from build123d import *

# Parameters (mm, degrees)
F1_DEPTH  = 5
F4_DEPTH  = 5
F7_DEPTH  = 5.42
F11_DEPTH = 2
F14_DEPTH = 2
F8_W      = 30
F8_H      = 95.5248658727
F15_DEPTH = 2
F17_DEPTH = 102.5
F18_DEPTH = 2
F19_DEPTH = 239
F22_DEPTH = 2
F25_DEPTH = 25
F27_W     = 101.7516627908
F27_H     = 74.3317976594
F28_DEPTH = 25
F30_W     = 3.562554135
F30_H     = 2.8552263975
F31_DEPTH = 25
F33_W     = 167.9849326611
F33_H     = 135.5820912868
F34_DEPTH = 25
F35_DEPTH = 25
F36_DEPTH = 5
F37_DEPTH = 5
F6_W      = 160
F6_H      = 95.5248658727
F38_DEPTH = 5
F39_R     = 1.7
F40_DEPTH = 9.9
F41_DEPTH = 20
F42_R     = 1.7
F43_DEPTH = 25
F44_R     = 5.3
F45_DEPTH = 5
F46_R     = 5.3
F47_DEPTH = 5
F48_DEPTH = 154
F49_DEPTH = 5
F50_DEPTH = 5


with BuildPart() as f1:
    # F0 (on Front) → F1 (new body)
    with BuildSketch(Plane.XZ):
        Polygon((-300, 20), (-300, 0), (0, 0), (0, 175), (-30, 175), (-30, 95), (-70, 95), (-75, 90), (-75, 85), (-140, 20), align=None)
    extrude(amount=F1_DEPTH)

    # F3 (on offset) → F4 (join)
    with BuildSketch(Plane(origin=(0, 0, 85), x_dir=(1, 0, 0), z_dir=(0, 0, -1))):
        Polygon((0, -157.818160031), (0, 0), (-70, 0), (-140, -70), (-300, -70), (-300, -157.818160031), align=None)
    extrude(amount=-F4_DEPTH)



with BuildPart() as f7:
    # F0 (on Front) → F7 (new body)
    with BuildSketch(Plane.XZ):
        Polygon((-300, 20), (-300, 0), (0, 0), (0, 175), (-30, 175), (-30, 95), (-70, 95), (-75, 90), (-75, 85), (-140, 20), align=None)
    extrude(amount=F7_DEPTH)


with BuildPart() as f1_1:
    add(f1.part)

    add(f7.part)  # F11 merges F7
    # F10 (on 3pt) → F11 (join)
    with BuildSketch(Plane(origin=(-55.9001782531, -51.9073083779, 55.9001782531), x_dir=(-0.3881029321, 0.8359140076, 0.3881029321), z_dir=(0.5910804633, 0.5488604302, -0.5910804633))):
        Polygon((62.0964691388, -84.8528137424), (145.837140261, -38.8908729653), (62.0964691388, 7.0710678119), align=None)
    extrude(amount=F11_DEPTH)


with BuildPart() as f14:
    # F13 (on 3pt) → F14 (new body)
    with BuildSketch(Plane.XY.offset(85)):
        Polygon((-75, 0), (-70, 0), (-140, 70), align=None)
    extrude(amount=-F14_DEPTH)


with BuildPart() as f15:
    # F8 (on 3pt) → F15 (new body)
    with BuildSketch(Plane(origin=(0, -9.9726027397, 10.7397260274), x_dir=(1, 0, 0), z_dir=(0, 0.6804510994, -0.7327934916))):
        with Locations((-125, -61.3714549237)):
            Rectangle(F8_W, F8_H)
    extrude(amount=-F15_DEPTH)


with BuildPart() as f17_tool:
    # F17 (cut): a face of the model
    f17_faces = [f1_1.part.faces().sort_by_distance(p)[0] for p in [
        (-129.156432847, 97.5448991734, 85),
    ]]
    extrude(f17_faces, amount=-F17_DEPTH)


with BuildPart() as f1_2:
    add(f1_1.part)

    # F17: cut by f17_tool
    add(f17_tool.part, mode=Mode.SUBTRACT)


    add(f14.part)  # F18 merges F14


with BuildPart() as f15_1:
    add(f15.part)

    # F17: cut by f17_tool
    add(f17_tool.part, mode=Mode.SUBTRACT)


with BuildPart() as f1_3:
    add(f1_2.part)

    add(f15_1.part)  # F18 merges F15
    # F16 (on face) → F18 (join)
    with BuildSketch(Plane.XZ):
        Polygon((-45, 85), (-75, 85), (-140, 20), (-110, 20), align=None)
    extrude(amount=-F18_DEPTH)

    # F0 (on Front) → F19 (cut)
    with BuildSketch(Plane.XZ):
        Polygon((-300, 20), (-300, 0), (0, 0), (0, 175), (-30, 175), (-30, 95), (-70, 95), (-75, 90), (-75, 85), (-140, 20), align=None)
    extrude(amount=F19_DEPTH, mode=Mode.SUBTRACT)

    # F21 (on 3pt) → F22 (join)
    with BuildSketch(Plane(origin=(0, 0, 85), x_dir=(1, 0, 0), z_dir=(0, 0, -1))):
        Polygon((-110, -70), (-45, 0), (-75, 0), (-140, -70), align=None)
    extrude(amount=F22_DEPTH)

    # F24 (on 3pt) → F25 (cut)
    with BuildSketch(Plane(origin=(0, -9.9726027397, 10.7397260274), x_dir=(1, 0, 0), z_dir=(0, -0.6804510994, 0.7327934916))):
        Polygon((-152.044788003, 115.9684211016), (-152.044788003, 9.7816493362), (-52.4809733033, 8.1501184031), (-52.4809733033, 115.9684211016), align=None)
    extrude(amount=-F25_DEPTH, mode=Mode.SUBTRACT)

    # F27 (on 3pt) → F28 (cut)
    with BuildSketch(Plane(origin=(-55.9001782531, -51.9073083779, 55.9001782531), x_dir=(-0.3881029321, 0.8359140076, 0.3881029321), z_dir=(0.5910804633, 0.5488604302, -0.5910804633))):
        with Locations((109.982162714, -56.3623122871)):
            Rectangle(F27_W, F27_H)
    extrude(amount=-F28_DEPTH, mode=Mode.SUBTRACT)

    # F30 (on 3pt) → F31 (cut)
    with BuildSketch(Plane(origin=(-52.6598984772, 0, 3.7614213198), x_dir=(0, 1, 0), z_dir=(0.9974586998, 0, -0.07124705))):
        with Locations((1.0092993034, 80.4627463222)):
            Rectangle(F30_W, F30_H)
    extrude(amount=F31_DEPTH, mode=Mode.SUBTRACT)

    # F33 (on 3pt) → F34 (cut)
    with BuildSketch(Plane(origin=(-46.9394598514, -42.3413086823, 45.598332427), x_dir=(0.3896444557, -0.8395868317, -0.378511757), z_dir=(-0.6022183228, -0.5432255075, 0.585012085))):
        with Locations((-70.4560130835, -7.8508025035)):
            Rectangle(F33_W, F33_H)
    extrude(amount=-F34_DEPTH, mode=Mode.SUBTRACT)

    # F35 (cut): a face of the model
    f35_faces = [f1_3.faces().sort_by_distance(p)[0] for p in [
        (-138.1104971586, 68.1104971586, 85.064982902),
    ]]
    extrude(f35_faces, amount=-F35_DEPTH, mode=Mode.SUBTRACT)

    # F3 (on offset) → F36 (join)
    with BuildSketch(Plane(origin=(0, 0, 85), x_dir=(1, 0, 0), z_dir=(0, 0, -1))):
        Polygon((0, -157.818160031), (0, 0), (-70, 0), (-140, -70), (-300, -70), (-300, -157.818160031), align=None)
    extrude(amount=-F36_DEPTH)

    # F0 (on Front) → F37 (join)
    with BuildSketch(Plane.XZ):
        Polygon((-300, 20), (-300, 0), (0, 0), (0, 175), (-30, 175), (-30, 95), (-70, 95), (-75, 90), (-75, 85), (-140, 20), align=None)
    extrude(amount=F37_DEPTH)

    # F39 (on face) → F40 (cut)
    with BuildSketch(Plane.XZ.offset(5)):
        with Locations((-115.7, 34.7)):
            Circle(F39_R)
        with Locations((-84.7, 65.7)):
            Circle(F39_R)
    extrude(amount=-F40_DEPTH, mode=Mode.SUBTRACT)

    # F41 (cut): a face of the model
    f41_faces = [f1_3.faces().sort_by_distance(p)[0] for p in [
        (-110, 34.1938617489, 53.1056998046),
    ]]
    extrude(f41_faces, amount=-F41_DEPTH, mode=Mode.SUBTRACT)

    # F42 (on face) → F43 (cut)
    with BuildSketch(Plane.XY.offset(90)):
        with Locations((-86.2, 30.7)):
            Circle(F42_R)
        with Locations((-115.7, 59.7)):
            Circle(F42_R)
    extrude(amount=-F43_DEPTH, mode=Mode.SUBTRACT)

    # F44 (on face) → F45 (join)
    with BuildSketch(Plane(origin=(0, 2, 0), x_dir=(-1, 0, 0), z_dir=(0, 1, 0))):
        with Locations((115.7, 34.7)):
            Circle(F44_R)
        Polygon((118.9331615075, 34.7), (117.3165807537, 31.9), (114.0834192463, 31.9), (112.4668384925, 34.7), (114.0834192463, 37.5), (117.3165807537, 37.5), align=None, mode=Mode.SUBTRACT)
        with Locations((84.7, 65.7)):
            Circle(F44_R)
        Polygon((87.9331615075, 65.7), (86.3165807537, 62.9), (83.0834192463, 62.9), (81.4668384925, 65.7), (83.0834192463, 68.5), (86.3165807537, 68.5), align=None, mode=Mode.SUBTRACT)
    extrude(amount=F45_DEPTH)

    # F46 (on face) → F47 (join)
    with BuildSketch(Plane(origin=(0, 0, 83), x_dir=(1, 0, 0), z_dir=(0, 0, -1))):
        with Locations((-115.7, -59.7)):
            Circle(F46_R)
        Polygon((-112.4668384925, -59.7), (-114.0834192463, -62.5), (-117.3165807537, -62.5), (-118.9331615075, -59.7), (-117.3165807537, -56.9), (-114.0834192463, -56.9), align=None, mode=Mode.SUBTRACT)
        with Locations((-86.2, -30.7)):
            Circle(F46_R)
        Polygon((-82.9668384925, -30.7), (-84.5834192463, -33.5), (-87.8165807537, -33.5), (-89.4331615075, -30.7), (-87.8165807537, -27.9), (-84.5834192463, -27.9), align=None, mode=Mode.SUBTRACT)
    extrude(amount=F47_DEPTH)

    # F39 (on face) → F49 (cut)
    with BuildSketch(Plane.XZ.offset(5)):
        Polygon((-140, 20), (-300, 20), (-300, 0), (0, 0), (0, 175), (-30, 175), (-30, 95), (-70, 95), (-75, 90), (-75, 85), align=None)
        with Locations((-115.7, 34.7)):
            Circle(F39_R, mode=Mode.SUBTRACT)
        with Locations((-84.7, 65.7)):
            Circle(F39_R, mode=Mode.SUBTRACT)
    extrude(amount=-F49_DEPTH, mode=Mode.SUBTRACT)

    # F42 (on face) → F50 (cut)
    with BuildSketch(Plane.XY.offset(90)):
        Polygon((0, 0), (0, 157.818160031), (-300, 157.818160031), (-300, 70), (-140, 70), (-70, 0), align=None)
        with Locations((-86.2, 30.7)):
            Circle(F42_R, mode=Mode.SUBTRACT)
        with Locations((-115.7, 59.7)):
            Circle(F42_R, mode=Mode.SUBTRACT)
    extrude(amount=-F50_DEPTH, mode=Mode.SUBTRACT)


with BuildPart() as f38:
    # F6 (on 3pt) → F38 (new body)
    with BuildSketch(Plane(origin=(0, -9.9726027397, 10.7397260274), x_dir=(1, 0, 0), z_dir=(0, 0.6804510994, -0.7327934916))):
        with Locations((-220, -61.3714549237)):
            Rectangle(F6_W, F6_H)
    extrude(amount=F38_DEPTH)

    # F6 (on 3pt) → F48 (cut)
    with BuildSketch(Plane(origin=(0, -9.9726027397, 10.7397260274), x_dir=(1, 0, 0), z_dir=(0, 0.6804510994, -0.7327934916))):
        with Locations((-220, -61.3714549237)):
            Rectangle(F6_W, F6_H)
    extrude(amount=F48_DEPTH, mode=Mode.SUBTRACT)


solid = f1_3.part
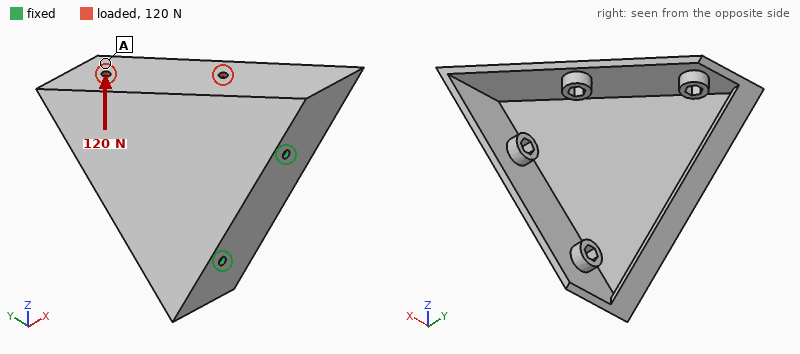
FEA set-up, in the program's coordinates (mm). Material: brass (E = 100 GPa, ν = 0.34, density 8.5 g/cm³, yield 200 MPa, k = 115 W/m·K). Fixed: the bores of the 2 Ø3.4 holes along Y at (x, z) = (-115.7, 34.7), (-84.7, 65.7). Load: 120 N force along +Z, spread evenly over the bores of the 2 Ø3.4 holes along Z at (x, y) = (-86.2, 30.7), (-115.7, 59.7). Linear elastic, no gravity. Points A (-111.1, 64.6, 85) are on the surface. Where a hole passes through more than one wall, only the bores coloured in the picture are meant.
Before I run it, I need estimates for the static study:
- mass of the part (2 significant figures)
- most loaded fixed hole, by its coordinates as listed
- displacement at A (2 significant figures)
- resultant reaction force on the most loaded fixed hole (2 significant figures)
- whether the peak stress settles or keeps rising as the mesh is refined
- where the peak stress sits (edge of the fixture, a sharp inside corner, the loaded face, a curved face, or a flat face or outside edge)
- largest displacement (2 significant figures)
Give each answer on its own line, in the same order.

140 g
(-84.7, 65.7)
0.76 mm
130 N
keeps rising
edge of the fixture
0.83 mm
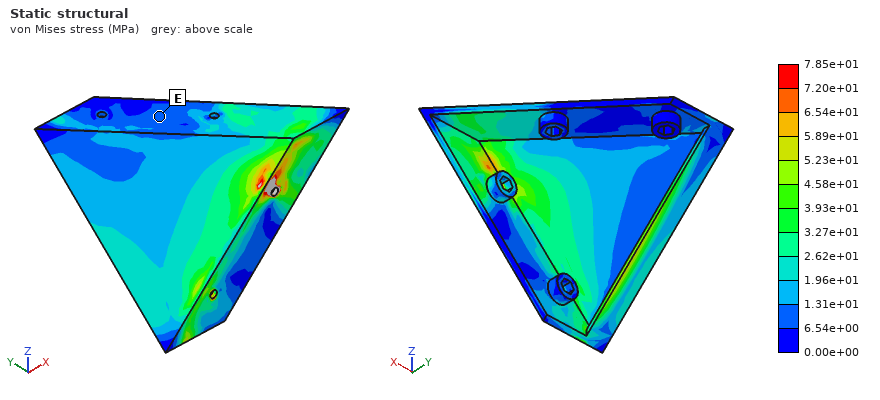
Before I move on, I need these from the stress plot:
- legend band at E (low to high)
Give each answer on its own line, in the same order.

6.54e+00 to 1.31e+01 MPa
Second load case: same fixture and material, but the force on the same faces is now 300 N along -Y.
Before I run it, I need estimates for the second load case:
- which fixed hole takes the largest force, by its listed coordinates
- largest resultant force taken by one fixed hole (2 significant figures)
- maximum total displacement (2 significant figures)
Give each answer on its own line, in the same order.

(-84.7, 65.7)
310 N
1.2 mm
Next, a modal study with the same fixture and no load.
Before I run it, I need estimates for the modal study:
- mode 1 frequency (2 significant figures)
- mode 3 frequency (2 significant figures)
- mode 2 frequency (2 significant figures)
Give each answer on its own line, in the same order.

260 Hz
1800 Hz
1000 Hz
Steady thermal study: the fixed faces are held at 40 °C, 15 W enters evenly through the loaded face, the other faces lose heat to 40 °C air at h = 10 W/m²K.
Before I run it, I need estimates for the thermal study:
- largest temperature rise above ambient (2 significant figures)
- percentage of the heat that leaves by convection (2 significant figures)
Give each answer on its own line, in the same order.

53 K
24 %
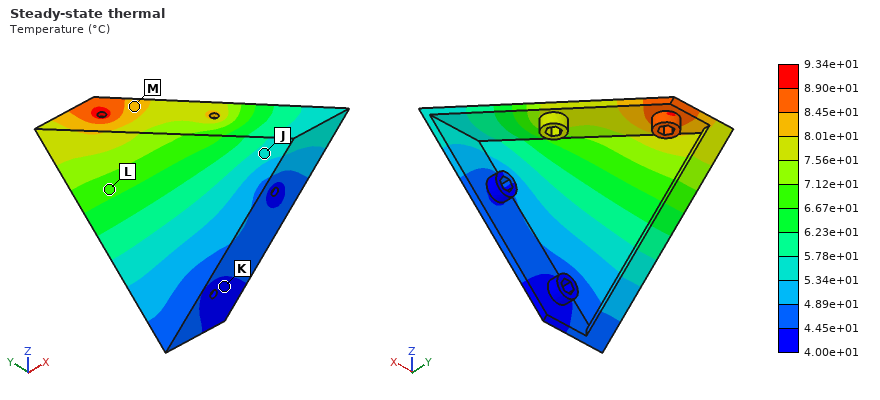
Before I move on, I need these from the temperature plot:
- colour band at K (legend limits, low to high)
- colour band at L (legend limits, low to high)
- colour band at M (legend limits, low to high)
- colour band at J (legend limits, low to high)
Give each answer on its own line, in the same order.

4.00e+01 to 4.45e+01 °C
6.67e+01 to 7.12e+01 °C
8.01e+01 to 8.45e+01 °C
5.34e+01 to 5.78e+01 °C
